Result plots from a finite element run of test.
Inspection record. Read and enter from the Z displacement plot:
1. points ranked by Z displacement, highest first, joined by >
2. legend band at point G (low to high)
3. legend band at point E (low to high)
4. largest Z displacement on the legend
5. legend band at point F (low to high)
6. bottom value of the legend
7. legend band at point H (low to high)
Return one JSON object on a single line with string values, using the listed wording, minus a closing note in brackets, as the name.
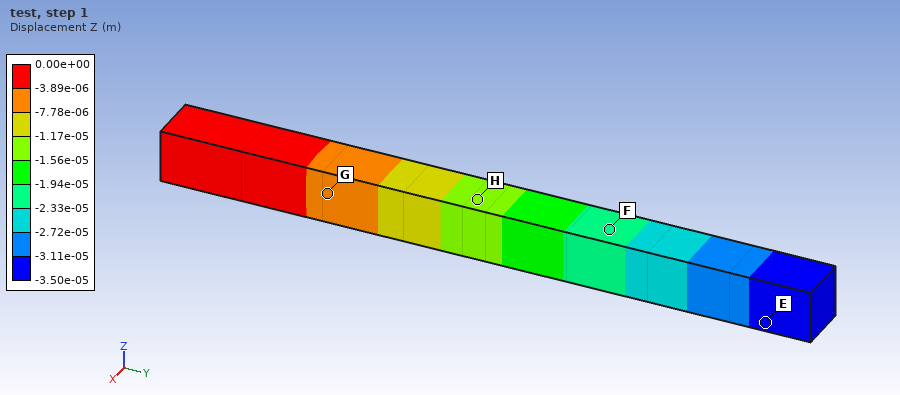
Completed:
{"points ranked by Z displacement, highest first, joined by >": "G > H > F > E", "legend band at point G": "-7.78e-06 to -3.89e-06 m", "legend band at point E": "-3.50e-05 to -3.11e-05 m", "largest Z displacement on the legend": "0.00e+00 m", "legend band at point F": "-2.33e-05 to -1.94e-05 m", "bottom value of the legend": "-3.50e-05 m", "legend band at point H": "-1.56e-05 to -1.17e-05 m"}
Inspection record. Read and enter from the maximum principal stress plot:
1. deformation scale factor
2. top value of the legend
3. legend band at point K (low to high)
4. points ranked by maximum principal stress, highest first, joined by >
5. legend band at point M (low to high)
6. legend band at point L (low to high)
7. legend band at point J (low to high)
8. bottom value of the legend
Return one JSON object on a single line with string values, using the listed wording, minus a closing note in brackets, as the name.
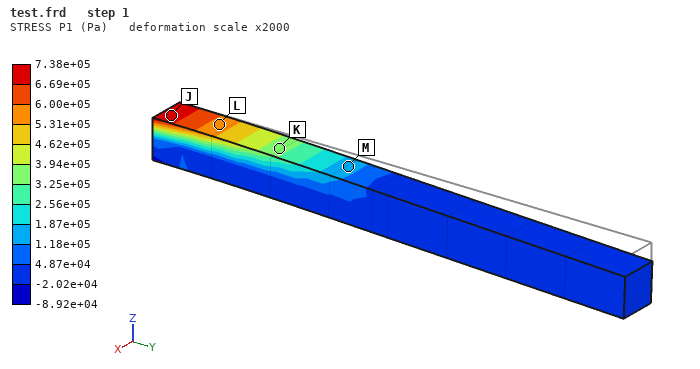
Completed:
{"deformation scale factor": "2000", "top value of the legend": "7.38e+05 Pa", "legend band at point K": "3.25e+05 to 3.94e+05 Pa", "points ranked by maximum principal stress, highest first, joined by >": "J > L > K > M", "legend band at point M": "1.18e+05 to 1.87e+05 Pa", "legend band at point L": "5.31e+05 to 6.00e+05 Pa", "legend band at point J": "6.69e+05 to 7.38e+05 Pa", "bottom value of the legend": "-8.92e+04 Pa"}
